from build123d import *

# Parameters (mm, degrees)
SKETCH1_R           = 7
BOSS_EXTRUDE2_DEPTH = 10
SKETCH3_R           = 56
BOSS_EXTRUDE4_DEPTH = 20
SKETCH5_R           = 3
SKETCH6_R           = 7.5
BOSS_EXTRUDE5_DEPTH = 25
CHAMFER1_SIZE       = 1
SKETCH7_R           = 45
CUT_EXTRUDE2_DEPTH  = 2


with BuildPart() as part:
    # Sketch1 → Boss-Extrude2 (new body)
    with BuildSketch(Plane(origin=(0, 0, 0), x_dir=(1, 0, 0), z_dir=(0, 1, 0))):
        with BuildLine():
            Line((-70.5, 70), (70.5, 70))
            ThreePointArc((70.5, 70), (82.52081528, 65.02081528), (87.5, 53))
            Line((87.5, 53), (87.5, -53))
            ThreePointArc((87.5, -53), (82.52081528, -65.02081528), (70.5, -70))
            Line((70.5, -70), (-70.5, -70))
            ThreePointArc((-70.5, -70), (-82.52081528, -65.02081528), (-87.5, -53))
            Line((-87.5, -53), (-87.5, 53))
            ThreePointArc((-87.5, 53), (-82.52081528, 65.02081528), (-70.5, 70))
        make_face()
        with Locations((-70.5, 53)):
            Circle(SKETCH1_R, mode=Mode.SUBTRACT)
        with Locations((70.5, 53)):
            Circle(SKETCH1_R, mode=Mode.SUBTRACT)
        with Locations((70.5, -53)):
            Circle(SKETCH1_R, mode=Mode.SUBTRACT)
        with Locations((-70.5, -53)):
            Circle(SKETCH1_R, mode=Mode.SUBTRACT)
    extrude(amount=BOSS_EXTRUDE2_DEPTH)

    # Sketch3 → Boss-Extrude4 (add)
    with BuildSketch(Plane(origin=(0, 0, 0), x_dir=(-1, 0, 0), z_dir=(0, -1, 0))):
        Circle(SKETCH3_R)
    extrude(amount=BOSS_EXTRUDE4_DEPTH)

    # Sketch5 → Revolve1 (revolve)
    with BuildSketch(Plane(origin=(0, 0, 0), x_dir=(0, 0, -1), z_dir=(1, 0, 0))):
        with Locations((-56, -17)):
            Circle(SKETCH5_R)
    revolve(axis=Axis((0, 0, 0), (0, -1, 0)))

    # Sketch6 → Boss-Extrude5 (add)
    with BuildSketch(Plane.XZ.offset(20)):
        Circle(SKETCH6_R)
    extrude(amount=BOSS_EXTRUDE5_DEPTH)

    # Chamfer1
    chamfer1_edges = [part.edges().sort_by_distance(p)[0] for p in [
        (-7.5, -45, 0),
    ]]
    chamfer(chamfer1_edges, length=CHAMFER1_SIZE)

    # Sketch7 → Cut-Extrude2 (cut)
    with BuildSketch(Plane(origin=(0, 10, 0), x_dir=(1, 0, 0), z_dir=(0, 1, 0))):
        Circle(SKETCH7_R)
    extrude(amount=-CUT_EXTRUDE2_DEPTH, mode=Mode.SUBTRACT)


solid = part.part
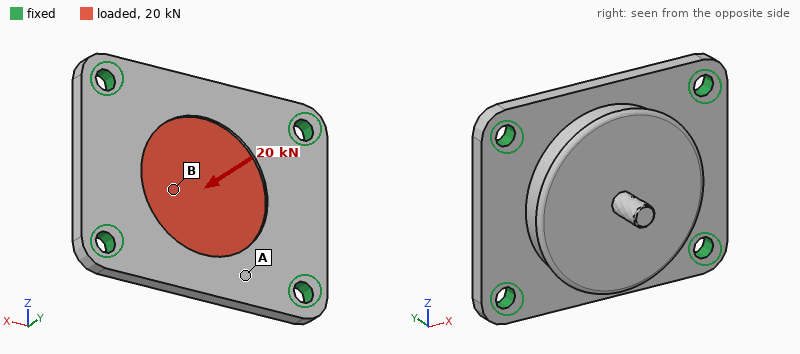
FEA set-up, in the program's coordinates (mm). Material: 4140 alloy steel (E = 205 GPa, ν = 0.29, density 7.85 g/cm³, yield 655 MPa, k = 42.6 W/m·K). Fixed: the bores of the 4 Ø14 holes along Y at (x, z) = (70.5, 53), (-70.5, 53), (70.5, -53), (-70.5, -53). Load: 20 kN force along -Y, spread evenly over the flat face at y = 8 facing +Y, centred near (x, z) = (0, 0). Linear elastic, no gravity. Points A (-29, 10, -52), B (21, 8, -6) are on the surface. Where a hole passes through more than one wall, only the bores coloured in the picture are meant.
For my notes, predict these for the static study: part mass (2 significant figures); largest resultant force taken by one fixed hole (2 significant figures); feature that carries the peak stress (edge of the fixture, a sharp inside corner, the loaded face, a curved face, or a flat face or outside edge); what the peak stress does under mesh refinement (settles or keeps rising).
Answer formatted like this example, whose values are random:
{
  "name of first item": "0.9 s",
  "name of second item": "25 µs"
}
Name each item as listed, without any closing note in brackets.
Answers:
{
  "part mass": "3.4 kg",
  "largest resultant force taken by one fixed hole": "6.1 kN",
  "feature that carries the peak stress": "edge of the fixture",
  "what the peak stress does under mesh refinement": "keeps rising"
}
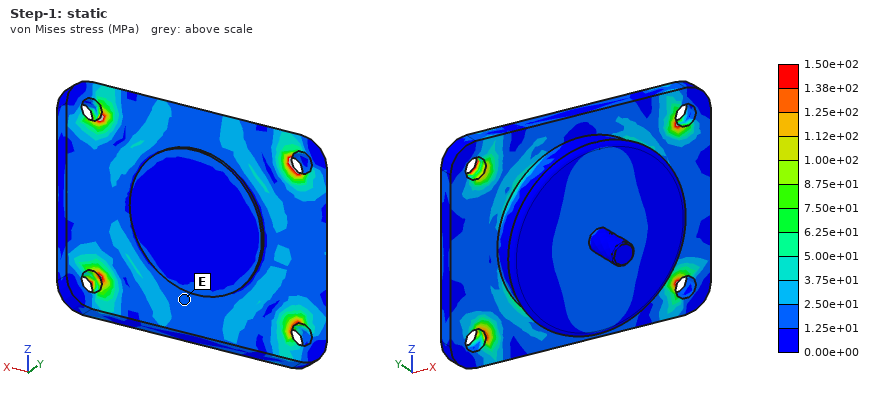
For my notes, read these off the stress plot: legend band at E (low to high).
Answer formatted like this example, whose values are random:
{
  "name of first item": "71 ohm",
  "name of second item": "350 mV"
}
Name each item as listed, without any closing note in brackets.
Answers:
{
  "legend band at E": "1.25e+01 to 2.50e+01 MPa"
}
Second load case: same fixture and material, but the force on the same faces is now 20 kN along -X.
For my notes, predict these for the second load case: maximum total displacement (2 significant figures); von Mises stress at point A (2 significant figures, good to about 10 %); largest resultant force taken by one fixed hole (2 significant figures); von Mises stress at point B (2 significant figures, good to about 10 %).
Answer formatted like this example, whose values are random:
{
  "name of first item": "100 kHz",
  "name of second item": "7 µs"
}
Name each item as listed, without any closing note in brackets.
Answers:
{
  "maximum total displacement": "4.2 µm",
  "von Mises stress at point A": "10 MPa",
  "largest resultant force taken by one fixed hole": "5.2 kN",
  "von Mises stress at point B": "6.4 MPa"
}
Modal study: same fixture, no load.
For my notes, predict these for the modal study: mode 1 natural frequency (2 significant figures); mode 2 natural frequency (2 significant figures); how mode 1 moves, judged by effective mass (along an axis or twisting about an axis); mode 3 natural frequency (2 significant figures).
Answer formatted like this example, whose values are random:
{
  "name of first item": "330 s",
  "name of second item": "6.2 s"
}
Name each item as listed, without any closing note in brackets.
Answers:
{
  "mode 1 natural frequency": "2600 Hz",
  "mode 2 natural frequency": "3300 Hz",
  "how mode 1 moves, judged by effective mass": "along Y",
  "mode 3 natural frequency": "4500 Hz"
}
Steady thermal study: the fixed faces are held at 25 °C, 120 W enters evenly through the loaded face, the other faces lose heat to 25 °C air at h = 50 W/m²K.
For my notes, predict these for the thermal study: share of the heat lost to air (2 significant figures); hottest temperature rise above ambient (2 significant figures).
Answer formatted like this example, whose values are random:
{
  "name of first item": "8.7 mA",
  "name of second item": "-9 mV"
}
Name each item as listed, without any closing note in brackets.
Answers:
{
  "share of the heat lost to air": "47 %",
  "hottest temperature rise above ambient": "41 K"
}
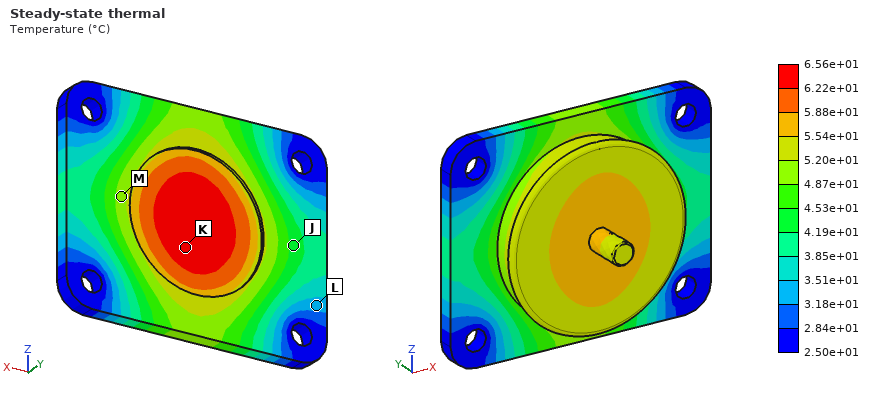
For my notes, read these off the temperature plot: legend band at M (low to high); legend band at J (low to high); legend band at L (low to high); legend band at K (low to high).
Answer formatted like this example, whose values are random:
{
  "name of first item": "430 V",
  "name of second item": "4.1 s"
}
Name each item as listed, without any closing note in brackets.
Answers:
{
  "legend band at M": "4.87e+01 to 5.20e+01 °C",
  "legend band at J": "4.19e+01 to 4.53e+01 °C",
  "legend band at L": "3.18e+01 to 3.51e+01 °C",
  "legend band at K": "6.22e+01 to 6.56e+01 °C"
}
